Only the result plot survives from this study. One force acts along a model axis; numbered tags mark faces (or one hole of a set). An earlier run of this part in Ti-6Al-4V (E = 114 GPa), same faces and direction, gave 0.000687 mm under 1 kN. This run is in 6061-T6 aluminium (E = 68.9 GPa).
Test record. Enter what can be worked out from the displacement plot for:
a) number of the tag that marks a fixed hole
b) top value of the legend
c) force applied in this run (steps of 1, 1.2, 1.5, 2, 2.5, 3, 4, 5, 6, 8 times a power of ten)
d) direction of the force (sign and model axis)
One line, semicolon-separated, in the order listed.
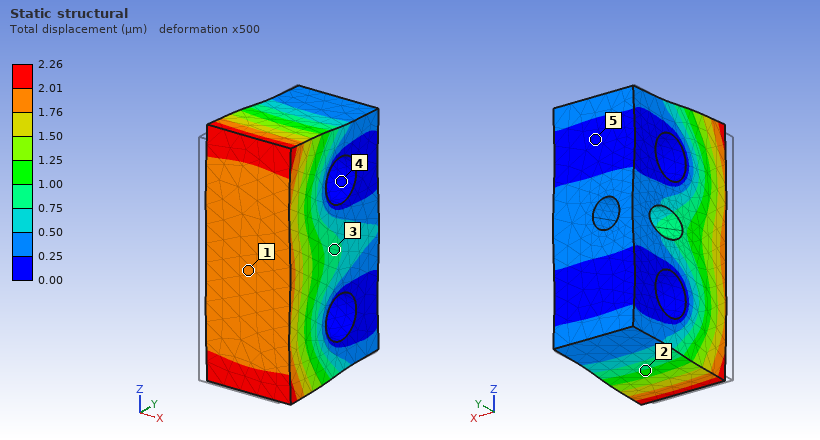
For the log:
4; 2.26 µm; 2 kN; +Y
